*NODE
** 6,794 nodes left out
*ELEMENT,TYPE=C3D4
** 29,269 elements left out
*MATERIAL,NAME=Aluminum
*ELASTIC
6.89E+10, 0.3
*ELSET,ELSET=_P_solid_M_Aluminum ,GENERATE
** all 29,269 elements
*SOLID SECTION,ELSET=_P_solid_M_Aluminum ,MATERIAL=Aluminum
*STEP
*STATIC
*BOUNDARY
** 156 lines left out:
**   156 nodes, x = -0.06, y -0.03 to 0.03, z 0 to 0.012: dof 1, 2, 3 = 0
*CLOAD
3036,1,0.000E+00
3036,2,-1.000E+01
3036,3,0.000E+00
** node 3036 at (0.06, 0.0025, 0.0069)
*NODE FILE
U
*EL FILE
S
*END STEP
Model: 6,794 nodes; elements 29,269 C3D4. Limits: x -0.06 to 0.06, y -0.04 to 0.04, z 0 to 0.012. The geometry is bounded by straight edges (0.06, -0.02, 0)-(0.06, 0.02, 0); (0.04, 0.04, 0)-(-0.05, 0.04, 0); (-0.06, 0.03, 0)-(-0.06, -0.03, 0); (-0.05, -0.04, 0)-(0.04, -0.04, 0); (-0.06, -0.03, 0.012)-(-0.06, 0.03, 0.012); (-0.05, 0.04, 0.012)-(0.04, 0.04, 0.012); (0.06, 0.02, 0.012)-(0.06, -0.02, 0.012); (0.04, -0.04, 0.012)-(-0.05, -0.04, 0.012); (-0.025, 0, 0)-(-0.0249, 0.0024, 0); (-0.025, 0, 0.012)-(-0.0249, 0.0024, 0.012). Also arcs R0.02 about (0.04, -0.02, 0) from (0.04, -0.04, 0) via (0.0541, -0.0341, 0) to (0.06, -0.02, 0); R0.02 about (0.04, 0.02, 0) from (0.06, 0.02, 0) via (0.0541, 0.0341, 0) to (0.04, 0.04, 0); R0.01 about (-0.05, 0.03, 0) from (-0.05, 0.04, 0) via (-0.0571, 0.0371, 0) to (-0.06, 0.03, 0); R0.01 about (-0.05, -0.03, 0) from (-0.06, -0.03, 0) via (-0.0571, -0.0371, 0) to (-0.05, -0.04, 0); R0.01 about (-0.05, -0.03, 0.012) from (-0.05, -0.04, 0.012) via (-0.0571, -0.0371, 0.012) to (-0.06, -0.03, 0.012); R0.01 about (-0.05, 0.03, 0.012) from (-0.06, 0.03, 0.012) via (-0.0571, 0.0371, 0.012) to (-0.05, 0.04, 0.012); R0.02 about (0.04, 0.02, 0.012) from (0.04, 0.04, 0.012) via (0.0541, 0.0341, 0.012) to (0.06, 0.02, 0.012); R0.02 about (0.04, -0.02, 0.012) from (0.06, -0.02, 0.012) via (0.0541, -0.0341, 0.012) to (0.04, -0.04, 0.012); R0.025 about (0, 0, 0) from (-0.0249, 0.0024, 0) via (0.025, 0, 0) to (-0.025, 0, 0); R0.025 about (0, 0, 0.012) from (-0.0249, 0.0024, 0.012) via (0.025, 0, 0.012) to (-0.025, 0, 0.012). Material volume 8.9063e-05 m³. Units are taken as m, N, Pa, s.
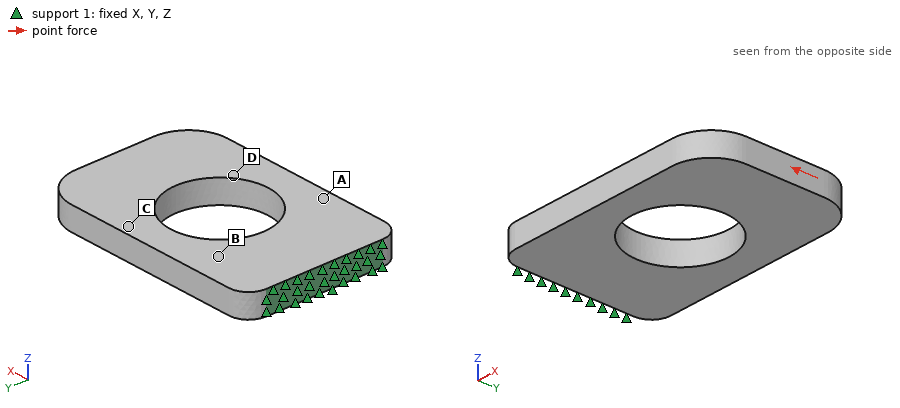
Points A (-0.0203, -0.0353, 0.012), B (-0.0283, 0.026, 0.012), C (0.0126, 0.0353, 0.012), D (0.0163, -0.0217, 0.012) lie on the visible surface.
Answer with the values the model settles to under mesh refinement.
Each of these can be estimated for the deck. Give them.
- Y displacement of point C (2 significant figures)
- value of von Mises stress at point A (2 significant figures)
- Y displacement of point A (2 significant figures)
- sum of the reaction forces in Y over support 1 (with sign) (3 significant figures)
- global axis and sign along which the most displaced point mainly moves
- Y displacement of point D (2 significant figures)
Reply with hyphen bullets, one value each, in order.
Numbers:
- -3.1e-07 m
- 1.0e+05 Pa
- -8.9e-08 m
- 10.0 N
- -Y
- -3.3e-07 m
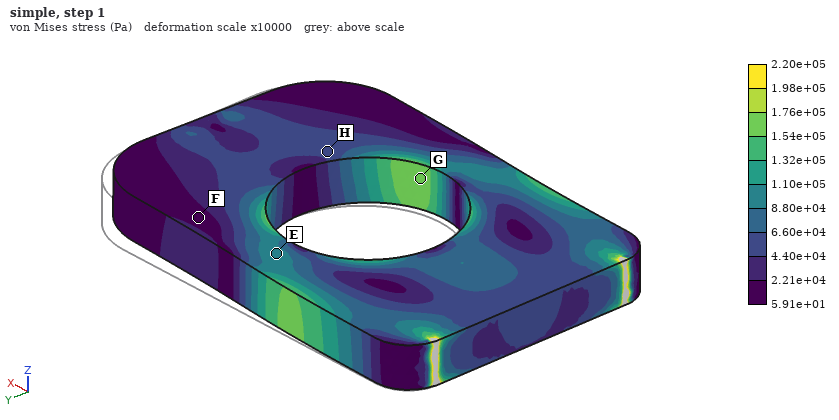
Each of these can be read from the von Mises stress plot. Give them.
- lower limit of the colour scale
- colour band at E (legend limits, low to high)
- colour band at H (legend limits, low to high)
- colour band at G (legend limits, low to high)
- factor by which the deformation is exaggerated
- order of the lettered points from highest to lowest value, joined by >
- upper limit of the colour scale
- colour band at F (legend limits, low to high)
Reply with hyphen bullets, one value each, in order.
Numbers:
- 5.91e+01 Pa
- 8.80e+04 to 1.10e+05 Pa
- 4.40e+04 to 6.60e+04 Pa
- 1.54e+05 to 1.76e+05 Pa
- 10000
- G > E > H > F
- 2.20e+05 Pa
- 5.91e+01 to 2.21e+04 Pa
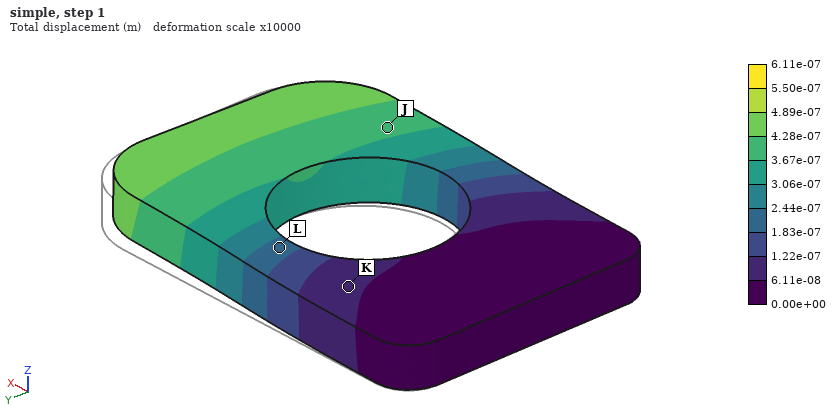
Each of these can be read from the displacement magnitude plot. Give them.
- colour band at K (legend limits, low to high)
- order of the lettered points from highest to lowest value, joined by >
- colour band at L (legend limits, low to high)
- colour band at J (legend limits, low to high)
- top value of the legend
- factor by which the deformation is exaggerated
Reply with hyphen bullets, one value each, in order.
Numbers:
- 6.11e-08 to 1.22e-07 m
- J > L > K
- 1.83e-07 to 2.44e-07 m
- 3.67e-07 to 4.28e-07 m
- 6.11e-07 m
- 10000
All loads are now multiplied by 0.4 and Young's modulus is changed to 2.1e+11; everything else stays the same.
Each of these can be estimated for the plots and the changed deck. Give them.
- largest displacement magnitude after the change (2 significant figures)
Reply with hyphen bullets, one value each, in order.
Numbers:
- 8.0e-08 m
